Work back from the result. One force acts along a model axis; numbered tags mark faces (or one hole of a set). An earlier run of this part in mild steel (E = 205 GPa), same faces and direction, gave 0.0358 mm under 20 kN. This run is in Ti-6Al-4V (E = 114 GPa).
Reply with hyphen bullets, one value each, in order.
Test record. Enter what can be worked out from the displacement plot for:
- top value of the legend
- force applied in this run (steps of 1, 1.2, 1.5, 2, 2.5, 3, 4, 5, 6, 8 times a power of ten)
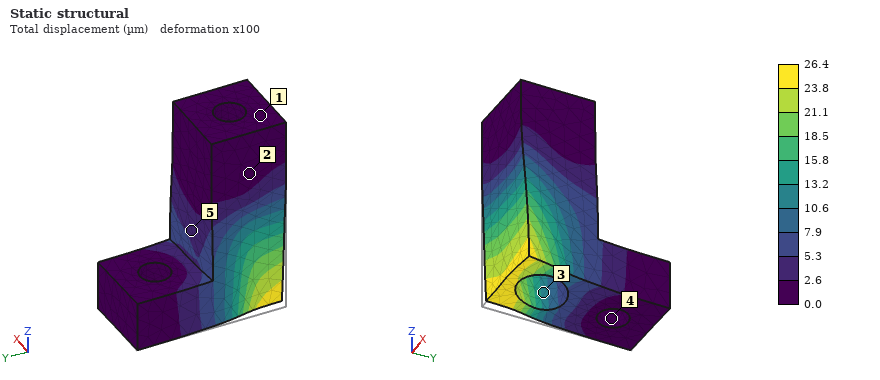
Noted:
- 26.4 µm
- 8 kN
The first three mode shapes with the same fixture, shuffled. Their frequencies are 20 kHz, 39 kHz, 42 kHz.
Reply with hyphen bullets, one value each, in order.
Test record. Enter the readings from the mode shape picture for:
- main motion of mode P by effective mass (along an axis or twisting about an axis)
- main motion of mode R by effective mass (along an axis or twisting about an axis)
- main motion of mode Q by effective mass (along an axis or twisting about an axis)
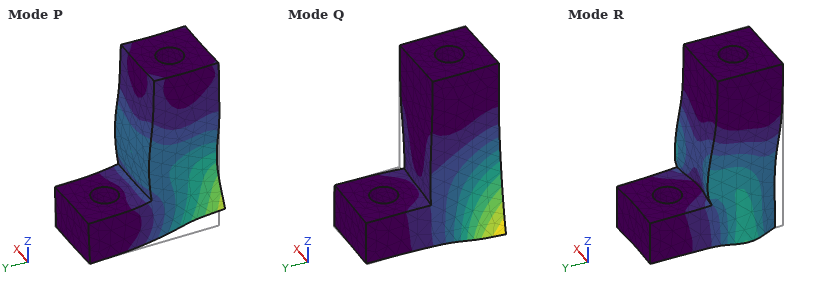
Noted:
- along Z
- along Y
- along X
